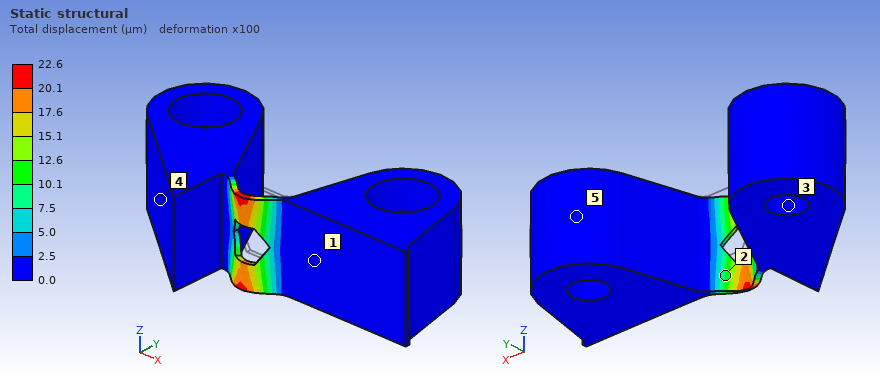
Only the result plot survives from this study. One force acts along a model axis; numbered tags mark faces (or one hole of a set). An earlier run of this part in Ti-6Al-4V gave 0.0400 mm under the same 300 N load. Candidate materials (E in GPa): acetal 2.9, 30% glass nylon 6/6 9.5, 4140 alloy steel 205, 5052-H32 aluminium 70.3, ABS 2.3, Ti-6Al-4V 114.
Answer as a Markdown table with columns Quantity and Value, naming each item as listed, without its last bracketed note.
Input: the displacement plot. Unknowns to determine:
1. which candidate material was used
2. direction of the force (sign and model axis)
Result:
| Quantity | Value |
|---|---|
| which candidate material was used | 4140 alloy steel |
| direction of the force | -Y |
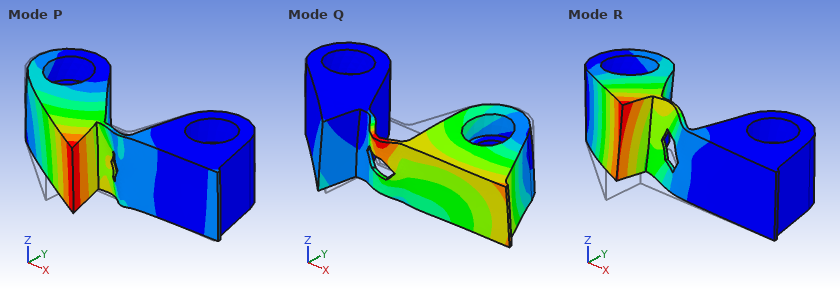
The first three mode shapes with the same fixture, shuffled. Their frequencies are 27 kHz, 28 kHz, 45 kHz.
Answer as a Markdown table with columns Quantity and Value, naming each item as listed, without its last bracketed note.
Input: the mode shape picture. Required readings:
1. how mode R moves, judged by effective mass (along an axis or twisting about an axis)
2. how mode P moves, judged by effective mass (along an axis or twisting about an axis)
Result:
| Quantity | Value |
|---|---|
| how mode R moves, judged by effective mass | along Z |
| how mode P moves, judged by effective mass | along X |
